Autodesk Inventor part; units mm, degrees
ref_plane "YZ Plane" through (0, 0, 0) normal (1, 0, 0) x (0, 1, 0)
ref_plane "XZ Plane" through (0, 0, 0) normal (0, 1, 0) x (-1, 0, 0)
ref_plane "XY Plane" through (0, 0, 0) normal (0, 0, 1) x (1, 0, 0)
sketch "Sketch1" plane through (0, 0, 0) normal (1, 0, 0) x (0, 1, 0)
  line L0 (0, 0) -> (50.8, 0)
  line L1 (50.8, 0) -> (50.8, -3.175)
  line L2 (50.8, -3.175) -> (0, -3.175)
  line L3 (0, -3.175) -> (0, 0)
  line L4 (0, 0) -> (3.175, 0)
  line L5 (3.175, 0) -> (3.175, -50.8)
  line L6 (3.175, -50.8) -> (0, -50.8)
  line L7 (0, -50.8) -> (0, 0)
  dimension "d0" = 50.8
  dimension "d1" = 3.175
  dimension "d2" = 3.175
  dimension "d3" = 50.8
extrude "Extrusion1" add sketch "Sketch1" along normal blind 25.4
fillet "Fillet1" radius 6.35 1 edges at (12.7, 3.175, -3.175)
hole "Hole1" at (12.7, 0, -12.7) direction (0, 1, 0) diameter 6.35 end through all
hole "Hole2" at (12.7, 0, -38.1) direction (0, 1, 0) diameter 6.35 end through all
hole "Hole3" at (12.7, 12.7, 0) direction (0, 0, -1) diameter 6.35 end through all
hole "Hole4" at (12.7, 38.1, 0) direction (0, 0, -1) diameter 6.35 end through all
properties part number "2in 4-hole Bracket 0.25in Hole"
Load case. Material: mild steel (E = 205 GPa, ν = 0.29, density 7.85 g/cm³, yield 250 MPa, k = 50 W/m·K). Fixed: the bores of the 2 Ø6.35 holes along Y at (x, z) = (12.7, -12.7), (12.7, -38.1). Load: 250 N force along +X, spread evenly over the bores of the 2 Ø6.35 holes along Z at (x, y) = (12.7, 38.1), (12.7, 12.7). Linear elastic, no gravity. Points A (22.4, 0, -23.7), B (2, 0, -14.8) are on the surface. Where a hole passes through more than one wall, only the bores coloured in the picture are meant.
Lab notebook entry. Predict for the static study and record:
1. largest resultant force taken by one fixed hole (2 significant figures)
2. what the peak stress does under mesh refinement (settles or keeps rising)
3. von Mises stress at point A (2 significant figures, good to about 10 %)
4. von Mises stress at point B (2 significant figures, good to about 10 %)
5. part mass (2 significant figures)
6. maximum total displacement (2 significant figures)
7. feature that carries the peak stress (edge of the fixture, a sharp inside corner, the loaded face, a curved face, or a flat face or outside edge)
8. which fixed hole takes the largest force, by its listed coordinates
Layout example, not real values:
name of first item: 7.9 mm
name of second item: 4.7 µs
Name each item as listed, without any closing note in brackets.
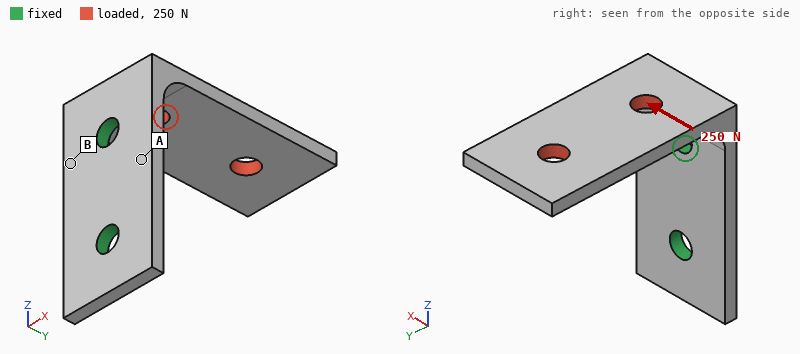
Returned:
largest resultant force taken by one fixed hole: 300 N
what the peak stress does under mesh refinement: keeps rising
von Mises stress at point A: 14 MPa
von Mises stress at point B: 37 MPa
part mass: 61 g
maximum total displacement: 70 µm
feature that carries the peak stress: edge of the fixture
which fixed hole takes the largest force, by its listed coordinates: (12.7, -12.7)
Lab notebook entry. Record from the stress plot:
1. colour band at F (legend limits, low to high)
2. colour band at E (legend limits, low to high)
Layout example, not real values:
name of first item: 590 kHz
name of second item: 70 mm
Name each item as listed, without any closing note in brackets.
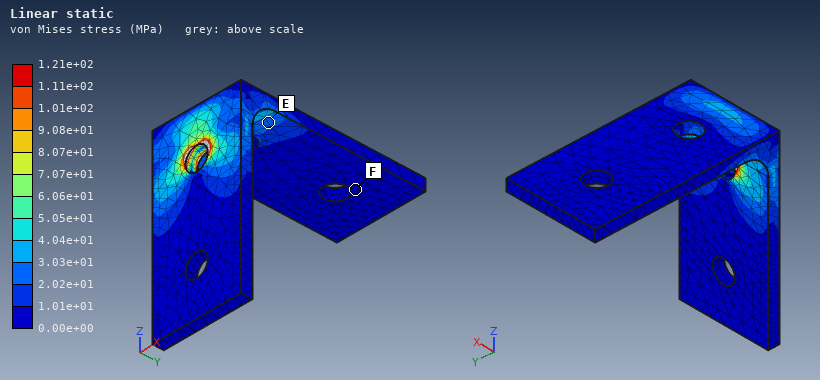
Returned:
colour band at F: 0.00e+00 to 1.01e+01 MPa
colour band at E: 2.02e+01 to 3.03e+01 MPa
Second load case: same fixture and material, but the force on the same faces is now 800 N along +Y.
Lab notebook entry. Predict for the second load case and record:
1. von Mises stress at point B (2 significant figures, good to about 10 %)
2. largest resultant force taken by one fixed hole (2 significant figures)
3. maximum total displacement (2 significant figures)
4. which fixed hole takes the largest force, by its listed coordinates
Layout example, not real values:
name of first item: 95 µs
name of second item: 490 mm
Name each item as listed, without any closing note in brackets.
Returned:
von Mises stress at point B: 36 MPa
largest resultant force taken by one fixed hole: 840 N
maximum total displacement: 0.11 mm
which fixed hole takes the largest force, by its listed coordinates: (12.7, -12.7)
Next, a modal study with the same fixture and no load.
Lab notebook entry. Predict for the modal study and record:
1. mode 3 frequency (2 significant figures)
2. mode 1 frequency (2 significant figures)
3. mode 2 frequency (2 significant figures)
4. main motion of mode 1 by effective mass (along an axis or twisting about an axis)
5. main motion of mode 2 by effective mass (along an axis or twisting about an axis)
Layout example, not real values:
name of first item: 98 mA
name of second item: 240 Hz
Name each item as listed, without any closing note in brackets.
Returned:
mode 3 frequency: 4500 Hz
mode 1 frequency: 990 Hz
mode 2 frequency: 2100 Hz
main motion of mode 1 by effective mass: along Z
main motion of mode 2 by effective mass: along X
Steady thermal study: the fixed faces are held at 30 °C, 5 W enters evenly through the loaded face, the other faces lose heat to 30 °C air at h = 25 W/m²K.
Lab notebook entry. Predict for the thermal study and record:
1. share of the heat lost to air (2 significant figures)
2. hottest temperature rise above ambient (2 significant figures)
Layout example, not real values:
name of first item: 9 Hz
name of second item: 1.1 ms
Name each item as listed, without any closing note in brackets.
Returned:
share of the heat lost to air: 30 %
hottest temperature rise above ambient: 29 K
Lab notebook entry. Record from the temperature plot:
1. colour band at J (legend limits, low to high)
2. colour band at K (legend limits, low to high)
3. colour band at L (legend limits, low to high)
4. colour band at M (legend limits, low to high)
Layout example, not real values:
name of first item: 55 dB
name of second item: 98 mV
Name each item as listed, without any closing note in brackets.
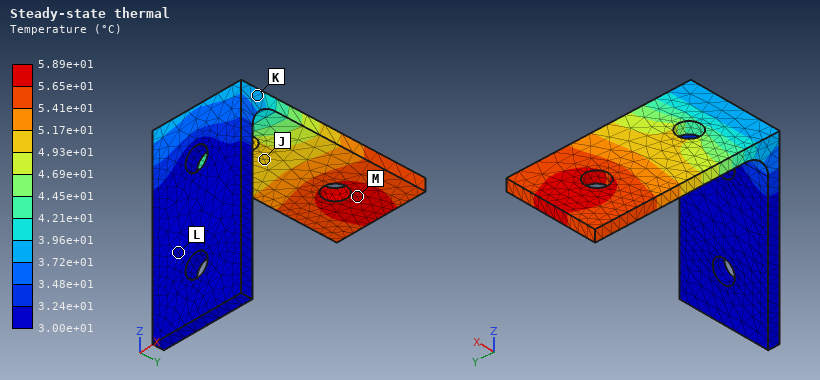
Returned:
colour band at J: 4.93e+01 to 5.17e+01 °C
colour band at K: 3.72e+01 to 3.96e+01 °C
colour band at L: 3.00e+01 to 3.24e+01 °C
colour band at M: 5.65e+01 to 5.89e+01 °C
